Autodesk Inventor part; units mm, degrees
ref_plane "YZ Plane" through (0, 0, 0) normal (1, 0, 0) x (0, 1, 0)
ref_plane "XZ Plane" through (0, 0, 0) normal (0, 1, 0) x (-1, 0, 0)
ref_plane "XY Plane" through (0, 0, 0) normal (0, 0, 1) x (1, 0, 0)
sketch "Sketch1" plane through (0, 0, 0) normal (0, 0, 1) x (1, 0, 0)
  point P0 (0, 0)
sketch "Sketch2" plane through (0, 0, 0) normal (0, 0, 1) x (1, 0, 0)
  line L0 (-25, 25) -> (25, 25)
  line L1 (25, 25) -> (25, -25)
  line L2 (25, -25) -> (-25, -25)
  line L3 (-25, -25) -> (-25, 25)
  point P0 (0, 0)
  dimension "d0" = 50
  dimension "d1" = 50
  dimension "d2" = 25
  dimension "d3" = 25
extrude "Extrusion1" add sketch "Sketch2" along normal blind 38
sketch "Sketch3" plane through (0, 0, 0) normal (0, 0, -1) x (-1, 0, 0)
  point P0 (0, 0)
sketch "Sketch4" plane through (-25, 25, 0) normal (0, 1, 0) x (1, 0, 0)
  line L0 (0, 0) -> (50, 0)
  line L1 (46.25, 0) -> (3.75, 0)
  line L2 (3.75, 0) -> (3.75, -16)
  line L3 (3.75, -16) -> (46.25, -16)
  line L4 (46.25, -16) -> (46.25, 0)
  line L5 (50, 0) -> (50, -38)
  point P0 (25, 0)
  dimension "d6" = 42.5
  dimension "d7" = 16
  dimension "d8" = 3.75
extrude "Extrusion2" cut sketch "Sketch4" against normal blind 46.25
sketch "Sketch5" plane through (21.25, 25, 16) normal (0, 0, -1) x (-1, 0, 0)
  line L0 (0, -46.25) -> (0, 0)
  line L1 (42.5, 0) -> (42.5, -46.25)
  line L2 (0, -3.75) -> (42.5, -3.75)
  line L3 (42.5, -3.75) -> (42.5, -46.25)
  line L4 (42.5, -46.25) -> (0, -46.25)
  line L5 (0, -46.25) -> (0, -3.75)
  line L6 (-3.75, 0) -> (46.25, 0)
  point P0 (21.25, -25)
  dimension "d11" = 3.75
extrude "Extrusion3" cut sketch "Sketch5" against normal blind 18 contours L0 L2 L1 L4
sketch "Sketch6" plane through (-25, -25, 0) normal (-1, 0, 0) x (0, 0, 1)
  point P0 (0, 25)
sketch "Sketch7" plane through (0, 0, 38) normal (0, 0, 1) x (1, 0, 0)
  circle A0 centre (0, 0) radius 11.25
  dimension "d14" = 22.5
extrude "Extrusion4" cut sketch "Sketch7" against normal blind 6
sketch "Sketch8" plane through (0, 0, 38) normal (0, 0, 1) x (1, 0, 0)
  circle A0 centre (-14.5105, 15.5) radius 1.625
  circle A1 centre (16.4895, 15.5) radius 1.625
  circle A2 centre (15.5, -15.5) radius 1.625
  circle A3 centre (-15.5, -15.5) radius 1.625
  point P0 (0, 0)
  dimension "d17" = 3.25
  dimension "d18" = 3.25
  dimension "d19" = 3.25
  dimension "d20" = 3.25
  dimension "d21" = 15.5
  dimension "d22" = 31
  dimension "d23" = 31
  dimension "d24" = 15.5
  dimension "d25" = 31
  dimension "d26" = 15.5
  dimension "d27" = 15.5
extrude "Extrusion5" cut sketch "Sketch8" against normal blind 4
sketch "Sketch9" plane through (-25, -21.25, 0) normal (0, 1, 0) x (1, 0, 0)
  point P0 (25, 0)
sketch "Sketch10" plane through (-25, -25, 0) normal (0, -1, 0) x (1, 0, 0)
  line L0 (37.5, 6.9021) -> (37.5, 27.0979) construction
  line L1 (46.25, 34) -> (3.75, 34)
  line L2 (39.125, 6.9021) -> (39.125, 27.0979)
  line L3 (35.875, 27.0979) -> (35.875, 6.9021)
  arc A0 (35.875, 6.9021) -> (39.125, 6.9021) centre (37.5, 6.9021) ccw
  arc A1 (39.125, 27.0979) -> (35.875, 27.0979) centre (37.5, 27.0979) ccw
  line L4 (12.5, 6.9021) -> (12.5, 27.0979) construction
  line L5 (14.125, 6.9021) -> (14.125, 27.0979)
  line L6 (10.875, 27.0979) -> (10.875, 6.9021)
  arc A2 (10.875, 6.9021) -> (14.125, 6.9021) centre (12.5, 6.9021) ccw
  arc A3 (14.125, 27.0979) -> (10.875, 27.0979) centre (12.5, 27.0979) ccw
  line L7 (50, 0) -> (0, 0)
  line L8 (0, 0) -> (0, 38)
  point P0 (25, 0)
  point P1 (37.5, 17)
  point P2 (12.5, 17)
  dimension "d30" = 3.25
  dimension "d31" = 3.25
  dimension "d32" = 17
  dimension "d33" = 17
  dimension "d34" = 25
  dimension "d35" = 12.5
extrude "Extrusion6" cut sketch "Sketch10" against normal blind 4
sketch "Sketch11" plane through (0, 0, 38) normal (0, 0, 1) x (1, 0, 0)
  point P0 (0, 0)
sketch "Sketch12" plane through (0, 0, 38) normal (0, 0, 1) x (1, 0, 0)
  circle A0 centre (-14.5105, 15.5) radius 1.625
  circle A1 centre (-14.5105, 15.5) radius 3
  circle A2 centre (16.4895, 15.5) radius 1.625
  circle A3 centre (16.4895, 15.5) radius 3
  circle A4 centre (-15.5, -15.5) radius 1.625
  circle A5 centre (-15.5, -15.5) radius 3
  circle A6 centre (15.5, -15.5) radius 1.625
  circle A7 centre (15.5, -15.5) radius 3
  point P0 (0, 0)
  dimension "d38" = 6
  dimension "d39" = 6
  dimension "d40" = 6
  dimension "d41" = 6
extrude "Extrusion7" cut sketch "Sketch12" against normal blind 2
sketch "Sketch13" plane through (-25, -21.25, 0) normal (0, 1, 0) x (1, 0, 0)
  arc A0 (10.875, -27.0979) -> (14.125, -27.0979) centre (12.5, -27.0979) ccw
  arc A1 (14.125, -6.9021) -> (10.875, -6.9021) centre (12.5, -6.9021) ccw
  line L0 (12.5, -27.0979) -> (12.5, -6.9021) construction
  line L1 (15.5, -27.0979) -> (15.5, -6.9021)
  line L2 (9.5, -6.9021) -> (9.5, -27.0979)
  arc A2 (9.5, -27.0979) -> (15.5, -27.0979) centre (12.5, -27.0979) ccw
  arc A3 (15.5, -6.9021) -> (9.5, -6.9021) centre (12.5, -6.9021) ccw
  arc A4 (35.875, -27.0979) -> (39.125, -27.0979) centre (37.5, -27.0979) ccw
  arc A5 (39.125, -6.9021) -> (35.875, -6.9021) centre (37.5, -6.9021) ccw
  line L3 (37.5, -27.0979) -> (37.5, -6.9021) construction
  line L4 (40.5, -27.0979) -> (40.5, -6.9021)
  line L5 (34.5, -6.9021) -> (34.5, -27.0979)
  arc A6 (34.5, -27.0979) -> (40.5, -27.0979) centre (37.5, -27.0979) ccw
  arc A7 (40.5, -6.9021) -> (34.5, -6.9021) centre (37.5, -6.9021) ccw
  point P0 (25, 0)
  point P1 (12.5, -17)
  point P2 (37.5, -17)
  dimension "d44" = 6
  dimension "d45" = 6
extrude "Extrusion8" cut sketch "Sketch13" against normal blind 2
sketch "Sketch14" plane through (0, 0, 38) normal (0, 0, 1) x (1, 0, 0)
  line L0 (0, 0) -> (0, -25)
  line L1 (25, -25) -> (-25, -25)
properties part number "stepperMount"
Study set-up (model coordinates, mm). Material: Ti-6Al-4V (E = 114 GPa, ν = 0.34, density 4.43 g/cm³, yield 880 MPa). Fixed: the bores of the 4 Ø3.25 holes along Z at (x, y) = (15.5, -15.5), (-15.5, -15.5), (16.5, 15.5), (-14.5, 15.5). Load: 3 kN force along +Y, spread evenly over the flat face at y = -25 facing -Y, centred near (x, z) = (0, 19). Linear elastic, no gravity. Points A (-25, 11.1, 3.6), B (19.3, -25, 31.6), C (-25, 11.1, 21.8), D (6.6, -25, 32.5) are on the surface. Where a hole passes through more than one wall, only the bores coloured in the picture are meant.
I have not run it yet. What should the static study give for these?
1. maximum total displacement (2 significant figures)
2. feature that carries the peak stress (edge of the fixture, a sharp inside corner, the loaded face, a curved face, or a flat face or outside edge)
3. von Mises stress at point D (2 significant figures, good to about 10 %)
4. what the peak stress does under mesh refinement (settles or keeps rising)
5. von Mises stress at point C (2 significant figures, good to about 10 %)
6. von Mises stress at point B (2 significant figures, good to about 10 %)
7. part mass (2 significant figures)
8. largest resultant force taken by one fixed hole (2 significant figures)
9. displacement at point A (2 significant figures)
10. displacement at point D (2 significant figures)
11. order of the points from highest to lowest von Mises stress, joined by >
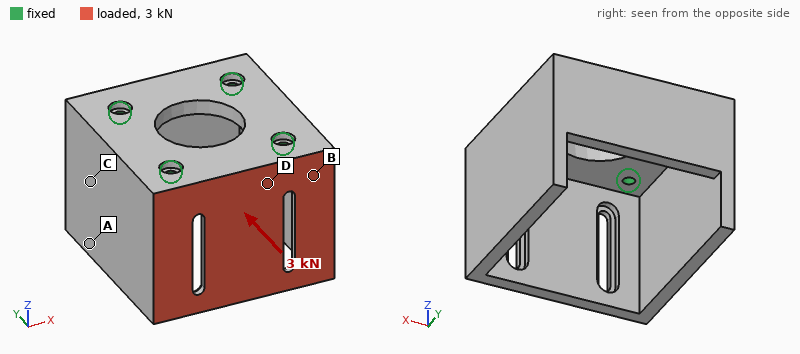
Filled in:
0.12 mm
edge of the fixture
59 MPa
keeps rising
20 MPa
38 MPa
130 g
1.4 kN
0.035 mm
0.023 mm
D > B > C > A
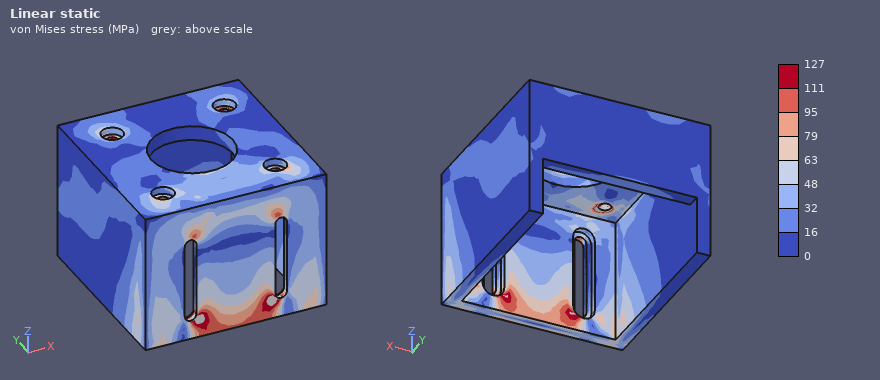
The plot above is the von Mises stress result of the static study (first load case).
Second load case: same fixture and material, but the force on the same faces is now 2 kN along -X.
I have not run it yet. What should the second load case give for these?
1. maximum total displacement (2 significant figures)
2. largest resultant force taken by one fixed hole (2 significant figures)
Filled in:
44 µm
1.5 kN
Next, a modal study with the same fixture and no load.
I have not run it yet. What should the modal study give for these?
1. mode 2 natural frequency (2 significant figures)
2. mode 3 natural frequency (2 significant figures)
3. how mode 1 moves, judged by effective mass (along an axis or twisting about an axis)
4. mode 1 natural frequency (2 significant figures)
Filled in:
4700 Hz
5200 Hz
along X
4400 Hz
